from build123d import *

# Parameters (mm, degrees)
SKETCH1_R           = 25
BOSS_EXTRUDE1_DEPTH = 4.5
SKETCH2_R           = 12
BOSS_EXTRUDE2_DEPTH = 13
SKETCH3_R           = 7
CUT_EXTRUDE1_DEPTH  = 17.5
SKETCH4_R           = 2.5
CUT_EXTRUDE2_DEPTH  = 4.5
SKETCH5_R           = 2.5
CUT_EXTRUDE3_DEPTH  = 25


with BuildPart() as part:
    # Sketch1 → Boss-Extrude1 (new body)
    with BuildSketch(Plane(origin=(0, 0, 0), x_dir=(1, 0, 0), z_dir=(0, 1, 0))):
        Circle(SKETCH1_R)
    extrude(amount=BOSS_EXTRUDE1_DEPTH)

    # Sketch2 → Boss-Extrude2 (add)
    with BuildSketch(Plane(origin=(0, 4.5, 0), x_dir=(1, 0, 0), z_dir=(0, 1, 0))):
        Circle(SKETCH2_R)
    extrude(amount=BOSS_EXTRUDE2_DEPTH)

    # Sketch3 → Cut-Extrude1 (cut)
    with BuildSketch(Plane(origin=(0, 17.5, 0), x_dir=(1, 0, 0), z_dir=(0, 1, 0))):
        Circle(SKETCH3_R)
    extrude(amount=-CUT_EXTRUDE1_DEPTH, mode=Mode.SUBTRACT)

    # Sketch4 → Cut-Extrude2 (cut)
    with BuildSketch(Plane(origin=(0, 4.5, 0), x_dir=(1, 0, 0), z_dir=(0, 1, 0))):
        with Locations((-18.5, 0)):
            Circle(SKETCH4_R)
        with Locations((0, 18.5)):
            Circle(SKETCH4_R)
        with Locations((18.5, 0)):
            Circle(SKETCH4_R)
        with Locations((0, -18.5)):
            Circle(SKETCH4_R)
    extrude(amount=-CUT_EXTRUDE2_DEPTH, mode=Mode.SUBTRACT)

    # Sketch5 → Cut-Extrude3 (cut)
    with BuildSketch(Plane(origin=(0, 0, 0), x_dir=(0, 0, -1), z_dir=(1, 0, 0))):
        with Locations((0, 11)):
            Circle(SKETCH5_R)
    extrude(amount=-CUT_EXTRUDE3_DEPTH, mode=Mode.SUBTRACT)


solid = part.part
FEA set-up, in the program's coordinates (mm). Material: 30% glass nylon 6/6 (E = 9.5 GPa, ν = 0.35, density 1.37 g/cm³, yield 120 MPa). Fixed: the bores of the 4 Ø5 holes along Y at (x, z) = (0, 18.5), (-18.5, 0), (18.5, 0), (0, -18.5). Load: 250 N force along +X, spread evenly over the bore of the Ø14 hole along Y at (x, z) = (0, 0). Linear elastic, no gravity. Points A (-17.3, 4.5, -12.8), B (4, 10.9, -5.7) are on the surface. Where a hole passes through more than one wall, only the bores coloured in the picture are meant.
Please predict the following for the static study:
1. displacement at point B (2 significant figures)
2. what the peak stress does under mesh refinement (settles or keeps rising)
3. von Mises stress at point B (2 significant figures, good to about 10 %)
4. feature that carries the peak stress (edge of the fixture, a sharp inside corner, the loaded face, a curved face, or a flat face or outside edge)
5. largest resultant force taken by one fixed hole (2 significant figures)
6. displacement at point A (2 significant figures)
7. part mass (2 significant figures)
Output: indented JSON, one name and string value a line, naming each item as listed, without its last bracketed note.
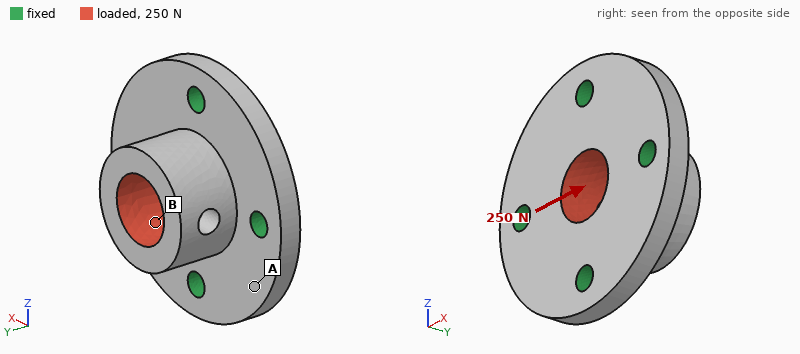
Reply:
{
  "displacement at point B": "4.5 µm",
  "what the peak stress does under mesh refinement": "keeps rising",
  "von Mises stress at point B": "1.3 MPa",
  "feature that carries the peak stress": "edge of the fixture",
  "largest resultant force taken by one fixed hole": "94 N",
  "displacement at point A": "1.3 µm",
  "part mass": "16 g"
}
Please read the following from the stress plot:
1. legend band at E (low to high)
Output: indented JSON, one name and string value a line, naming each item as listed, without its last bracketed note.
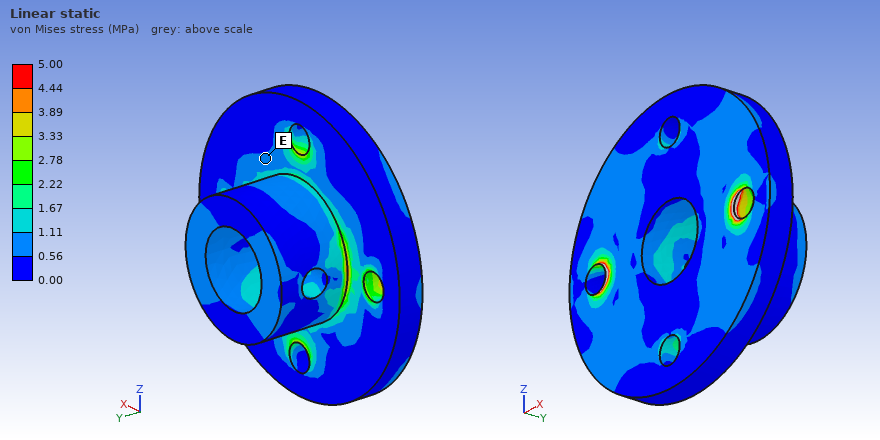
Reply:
{
  "legend band at E": "0.56 to 1.11 MPa"
}
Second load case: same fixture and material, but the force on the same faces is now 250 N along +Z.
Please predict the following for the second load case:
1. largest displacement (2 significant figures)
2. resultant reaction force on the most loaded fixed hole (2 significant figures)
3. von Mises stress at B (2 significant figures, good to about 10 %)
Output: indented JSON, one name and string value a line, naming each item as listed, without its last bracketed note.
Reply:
{
  "largest displacement": "7.8 µm",
  "resultant reaction force on the most loaded fixed hole": "93 N",
  "von Mises stress at B": "1.1 MPa"
}
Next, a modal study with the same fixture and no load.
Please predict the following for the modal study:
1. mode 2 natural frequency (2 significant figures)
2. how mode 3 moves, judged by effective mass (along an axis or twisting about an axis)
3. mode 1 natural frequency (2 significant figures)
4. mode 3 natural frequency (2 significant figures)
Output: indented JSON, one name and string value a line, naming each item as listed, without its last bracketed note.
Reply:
{
  "mode 2 natural frequency": "11 kHz",
  "how mode 3 moves, judged by effective mass": "along Y",
  "mode 1 natural frequency": "11 kHz",
  "mode 3 natural frequency": "12 kHz"
}
